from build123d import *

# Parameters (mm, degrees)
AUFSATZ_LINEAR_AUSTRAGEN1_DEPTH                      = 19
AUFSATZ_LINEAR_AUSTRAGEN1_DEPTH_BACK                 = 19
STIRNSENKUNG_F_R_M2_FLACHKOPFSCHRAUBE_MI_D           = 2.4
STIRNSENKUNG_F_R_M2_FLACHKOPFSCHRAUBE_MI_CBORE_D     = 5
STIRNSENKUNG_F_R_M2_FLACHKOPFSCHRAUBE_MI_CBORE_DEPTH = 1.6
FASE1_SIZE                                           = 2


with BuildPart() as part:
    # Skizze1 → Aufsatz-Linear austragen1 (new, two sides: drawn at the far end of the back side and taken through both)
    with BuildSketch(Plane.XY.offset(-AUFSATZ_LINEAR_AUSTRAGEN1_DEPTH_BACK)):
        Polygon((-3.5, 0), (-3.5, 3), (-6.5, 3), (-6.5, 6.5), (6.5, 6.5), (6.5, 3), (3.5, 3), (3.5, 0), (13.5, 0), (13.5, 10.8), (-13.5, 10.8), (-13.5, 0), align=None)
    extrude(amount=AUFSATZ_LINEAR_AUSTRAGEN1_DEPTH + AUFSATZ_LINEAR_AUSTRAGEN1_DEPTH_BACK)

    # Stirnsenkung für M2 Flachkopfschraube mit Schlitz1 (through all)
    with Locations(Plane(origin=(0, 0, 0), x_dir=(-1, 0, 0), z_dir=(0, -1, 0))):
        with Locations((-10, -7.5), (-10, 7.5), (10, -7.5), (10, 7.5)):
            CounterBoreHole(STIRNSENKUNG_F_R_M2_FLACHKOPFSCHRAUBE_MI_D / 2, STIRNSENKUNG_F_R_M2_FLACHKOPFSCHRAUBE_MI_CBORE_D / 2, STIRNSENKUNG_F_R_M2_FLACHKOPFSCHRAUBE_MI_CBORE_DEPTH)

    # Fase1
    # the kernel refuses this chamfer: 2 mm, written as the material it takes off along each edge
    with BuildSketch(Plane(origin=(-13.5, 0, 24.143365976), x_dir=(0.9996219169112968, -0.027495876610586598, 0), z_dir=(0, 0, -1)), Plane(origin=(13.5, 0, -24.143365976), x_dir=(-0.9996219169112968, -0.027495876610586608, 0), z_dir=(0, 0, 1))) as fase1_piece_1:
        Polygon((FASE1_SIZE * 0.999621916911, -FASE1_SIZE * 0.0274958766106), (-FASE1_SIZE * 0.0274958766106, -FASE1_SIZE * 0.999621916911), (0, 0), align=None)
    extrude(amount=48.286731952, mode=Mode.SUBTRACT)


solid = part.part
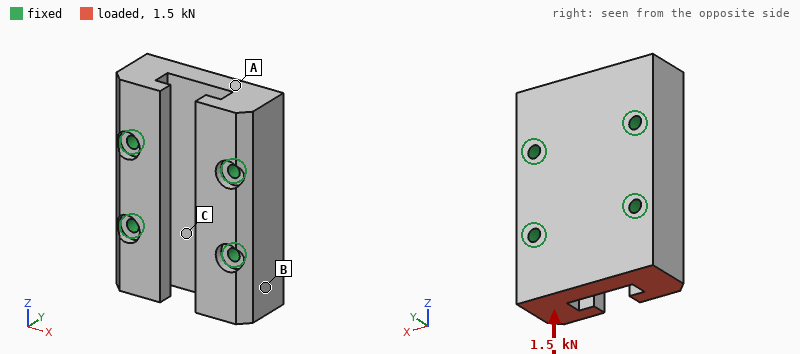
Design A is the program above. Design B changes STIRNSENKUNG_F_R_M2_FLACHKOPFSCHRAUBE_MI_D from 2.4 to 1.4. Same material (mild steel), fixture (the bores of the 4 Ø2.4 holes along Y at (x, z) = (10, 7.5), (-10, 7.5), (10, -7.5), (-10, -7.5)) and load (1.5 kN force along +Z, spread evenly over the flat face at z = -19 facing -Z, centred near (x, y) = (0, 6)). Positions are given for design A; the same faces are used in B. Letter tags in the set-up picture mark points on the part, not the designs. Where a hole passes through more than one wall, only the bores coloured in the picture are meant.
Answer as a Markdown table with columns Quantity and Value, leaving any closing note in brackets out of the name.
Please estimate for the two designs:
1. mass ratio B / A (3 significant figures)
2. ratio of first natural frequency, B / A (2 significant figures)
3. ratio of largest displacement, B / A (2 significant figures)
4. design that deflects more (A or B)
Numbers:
| Quantity | Value |
|---|---|
| mass ratio B / A | 1.01 |
| ratio of first natural frequency, B / A | 0.90 |
| ratio of largest displacement, B / A | 1.1 |
| design that deflects more | B |
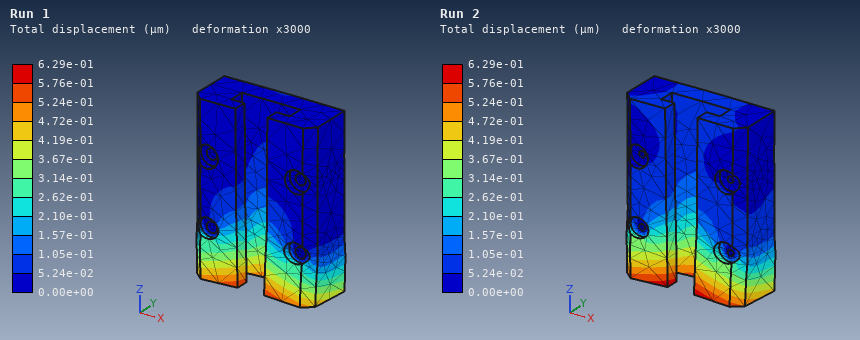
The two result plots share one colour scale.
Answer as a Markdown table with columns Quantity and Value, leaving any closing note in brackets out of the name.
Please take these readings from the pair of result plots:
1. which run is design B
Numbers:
| Quantity | Value |
|---|---|
| which run is design B | Run 2 |
